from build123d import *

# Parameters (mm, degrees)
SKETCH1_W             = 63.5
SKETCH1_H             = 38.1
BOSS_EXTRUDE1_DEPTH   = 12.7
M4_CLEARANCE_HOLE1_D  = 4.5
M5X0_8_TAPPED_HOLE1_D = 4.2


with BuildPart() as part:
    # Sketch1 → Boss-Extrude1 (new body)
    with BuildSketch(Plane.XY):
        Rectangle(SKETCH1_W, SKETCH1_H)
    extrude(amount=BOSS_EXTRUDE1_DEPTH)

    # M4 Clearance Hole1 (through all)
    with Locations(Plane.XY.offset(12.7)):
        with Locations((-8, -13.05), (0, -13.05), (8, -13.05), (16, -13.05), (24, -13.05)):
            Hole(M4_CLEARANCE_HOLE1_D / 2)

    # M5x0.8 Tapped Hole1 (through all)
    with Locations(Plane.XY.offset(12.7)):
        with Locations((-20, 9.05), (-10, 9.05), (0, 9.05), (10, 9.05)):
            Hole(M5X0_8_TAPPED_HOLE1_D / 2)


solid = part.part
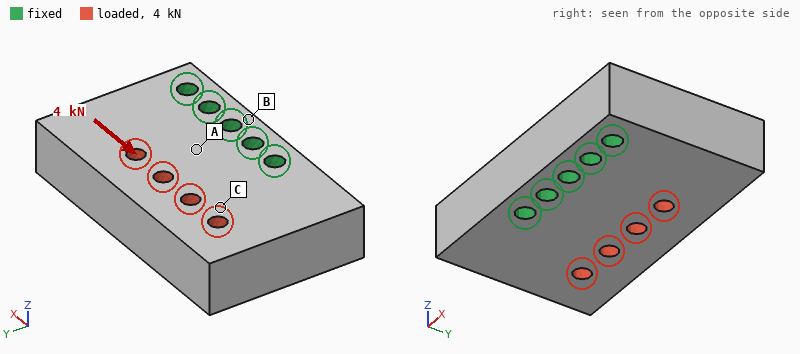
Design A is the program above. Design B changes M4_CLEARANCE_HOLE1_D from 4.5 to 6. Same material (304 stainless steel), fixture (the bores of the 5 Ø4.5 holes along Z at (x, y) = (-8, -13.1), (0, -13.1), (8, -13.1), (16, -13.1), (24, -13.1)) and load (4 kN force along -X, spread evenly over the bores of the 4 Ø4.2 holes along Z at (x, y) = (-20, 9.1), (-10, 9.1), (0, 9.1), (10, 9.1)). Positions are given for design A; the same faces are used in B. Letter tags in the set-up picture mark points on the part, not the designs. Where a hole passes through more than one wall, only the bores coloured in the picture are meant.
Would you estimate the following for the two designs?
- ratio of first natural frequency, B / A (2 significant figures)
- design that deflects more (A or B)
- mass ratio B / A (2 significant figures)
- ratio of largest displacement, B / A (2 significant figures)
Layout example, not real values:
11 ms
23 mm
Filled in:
1.1
A
0.97
0.90
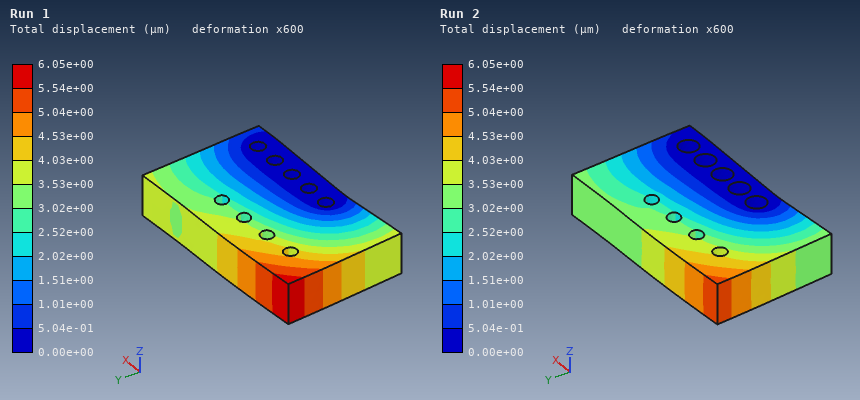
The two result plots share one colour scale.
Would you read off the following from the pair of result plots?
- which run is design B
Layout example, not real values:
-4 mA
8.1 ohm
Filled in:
Run 2
